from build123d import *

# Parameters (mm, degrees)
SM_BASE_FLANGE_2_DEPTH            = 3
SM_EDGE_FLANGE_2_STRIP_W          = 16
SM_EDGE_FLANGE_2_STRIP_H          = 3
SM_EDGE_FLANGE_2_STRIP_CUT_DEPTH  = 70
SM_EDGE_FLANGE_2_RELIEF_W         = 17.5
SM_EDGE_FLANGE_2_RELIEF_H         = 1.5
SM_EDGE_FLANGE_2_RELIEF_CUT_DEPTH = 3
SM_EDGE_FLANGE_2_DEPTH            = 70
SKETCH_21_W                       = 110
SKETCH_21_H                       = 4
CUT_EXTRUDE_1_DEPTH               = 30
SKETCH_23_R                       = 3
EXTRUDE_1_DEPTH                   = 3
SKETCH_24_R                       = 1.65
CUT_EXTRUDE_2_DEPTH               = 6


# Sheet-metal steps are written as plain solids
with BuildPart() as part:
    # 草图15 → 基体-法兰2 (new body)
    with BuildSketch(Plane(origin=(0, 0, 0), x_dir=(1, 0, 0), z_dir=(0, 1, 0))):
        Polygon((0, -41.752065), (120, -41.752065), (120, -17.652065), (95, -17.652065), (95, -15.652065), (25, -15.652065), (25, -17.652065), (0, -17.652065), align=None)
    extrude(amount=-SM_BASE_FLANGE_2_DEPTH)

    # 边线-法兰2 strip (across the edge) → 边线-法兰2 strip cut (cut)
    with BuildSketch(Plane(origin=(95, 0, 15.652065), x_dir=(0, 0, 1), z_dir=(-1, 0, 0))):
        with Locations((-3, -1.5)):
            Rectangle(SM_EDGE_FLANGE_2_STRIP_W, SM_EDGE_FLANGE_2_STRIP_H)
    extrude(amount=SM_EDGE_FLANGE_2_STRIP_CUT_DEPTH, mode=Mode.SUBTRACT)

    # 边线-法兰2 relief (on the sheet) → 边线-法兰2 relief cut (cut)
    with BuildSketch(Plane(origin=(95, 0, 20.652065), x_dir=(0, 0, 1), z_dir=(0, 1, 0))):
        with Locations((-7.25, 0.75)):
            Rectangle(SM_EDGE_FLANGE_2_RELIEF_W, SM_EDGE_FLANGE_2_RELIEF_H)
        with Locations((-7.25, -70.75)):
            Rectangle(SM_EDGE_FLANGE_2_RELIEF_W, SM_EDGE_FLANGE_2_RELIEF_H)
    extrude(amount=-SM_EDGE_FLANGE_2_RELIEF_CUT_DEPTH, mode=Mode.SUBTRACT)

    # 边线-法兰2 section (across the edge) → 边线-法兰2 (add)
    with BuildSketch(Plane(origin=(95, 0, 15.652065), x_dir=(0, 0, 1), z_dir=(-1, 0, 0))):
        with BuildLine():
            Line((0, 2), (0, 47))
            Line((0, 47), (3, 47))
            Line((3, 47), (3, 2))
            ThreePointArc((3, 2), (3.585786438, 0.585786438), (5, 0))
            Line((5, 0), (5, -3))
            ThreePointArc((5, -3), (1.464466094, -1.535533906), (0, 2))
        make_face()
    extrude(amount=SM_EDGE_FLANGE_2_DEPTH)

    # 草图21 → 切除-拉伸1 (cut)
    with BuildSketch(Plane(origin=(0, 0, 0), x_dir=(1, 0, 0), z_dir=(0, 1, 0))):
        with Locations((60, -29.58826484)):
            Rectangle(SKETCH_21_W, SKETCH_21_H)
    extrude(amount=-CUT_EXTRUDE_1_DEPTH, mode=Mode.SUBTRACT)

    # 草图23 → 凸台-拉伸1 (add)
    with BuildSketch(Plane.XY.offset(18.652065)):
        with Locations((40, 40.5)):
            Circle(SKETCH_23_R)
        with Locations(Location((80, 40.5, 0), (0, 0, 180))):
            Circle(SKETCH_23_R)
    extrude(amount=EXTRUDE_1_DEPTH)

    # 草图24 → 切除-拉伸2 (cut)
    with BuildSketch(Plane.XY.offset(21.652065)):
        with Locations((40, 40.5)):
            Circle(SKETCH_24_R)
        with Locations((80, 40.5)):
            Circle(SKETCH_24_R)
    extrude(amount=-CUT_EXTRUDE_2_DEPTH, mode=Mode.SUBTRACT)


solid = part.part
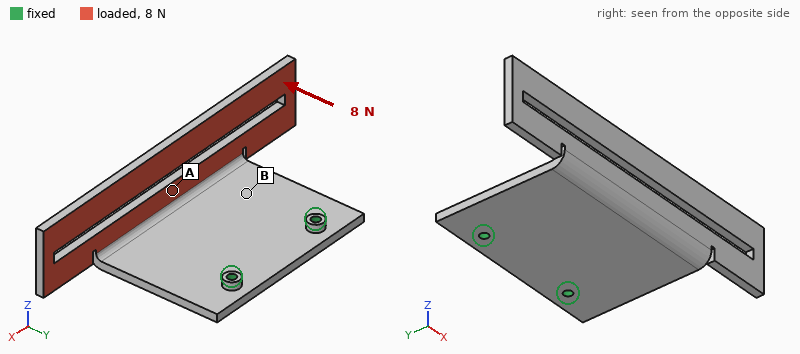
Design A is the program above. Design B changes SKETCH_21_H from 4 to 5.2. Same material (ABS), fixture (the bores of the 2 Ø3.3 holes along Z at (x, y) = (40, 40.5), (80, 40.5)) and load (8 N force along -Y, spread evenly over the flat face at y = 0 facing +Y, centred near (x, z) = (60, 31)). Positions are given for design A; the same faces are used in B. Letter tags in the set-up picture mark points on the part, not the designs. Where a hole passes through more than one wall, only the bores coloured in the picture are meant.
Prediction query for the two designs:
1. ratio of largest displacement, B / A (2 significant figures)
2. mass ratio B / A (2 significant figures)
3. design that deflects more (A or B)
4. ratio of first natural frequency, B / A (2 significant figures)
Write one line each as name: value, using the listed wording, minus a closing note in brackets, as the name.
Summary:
ratio of largest displacement, B / A: 1.1
mass ratio B / A: 0.98
design that deflects more: B
ratio of first natural frequency, B / A: 1.0
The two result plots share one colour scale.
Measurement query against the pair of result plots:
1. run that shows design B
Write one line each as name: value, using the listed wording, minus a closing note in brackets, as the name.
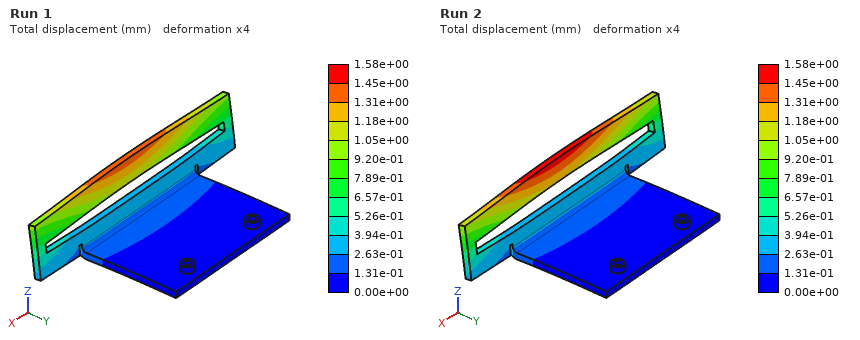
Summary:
run that shows design B: Run 2
